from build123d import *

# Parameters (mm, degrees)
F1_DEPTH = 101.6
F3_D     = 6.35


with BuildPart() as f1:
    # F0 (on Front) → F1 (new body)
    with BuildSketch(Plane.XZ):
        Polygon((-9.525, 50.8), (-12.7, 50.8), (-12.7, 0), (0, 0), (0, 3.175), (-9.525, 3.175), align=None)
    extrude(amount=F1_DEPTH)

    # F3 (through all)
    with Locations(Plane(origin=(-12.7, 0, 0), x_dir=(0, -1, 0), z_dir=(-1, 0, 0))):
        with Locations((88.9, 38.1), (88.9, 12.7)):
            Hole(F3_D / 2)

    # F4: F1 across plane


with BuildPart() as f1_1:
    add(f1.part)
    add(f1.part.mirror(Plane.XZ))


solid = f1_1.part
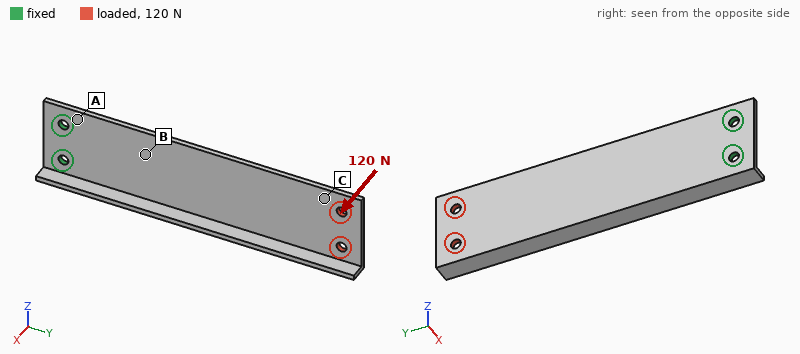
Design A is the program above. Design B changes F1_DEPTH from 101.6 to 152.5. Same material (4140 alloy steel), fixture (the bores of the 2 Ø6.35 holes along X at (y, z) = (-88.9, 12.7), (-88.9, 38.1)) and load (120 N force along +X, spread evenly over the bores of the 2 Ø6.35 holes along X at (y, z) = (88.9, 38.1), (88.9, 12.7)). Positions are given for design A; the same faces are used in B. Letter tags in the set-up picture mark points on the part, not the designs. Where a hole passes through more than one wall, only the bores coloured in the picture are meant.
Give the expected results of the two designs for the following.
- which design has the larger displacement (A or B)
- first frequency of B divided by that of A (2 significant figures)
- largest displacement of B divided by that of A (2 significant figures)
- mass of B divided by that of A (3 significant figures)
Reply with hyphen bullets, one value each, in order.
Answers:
- B
- 0.68
- 1.2
- 1.51
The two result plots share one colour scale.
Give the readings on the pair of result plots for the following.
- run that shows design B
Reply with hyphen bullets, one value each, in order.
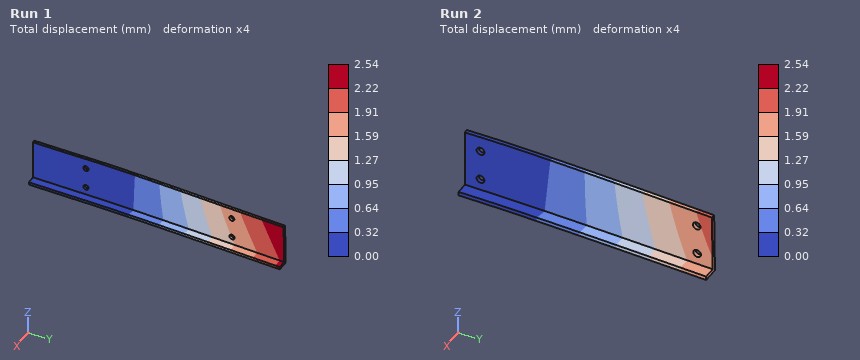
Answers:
- Run 1
